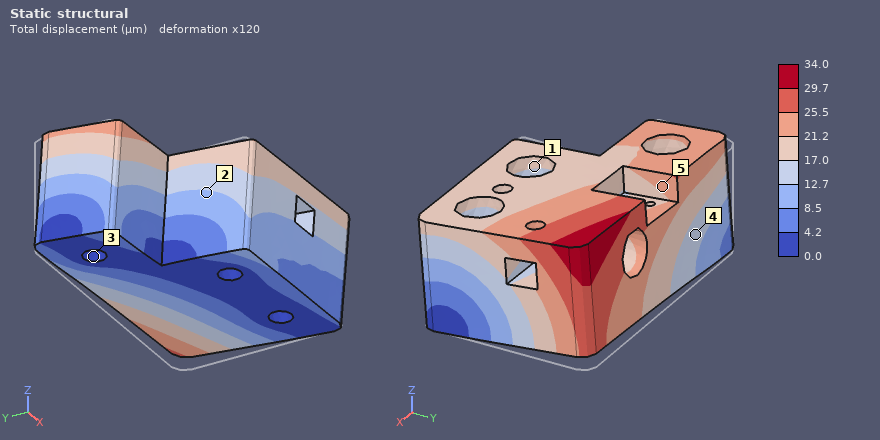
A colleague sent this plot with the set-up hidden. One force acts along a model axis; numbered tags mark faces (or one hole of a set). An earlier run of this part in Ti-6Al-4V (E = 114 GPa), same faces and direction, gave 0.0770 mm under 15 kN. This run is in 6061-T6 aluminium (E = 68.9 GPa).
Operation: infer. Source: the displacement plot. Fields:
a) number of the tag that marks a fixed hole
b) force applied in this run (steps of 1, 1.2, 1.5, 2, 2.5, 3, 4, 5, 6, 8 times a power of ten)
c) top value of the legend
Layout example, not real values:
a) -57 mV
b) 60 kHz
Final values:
a) 3
b) 4 kN
c) 34.0 µm
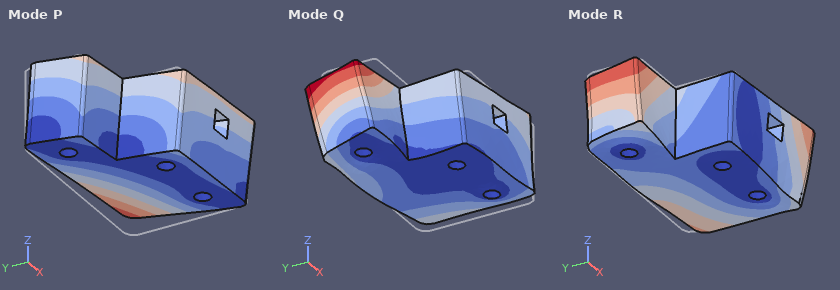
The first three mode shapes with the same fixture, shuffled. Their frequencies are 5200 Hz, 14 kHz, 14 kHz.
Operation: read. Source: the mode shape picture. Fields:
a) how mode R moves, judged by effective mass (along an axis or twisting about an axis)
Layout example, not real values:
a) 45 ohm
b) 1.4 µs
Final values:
a) along X
